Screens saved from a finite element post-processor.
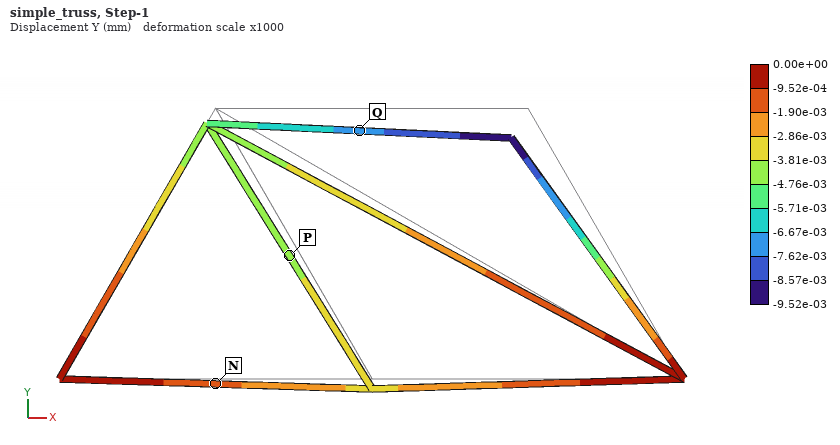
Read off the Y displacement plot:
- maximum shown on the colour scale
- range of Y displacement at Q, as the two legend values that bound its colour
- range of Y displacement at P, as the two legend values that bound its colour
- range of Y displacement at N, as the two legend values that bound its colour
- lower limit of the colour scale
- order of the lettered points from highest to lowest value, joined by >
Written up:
0.00e+00 mm
-7.62e-03 to -6.67e-03 mm
-4.76e-03 to -3.81e-03 mm
-1.90e-03 to -9.52e-04 mm
-9.52e-03 mm
N > P > Q
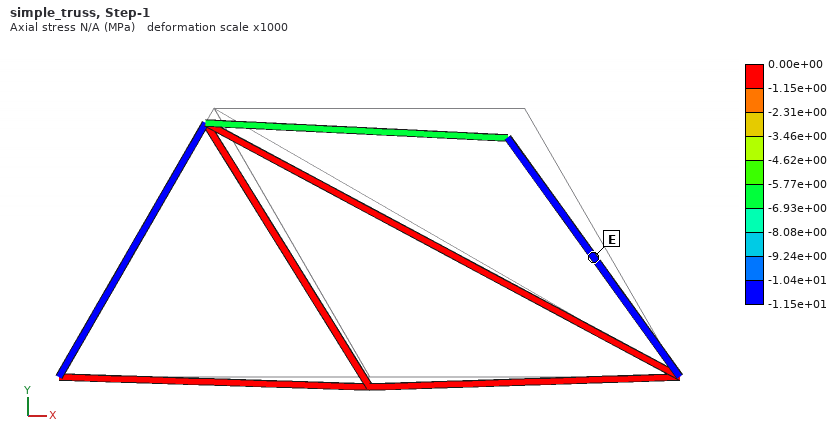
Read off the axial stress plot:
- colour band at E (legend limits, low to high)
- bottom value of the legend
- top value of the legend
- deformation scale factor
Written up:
-1.15e+01 to -1.04e+01 MPa
-1.15e+01 MPa
0.00e+00 MPa
1000
